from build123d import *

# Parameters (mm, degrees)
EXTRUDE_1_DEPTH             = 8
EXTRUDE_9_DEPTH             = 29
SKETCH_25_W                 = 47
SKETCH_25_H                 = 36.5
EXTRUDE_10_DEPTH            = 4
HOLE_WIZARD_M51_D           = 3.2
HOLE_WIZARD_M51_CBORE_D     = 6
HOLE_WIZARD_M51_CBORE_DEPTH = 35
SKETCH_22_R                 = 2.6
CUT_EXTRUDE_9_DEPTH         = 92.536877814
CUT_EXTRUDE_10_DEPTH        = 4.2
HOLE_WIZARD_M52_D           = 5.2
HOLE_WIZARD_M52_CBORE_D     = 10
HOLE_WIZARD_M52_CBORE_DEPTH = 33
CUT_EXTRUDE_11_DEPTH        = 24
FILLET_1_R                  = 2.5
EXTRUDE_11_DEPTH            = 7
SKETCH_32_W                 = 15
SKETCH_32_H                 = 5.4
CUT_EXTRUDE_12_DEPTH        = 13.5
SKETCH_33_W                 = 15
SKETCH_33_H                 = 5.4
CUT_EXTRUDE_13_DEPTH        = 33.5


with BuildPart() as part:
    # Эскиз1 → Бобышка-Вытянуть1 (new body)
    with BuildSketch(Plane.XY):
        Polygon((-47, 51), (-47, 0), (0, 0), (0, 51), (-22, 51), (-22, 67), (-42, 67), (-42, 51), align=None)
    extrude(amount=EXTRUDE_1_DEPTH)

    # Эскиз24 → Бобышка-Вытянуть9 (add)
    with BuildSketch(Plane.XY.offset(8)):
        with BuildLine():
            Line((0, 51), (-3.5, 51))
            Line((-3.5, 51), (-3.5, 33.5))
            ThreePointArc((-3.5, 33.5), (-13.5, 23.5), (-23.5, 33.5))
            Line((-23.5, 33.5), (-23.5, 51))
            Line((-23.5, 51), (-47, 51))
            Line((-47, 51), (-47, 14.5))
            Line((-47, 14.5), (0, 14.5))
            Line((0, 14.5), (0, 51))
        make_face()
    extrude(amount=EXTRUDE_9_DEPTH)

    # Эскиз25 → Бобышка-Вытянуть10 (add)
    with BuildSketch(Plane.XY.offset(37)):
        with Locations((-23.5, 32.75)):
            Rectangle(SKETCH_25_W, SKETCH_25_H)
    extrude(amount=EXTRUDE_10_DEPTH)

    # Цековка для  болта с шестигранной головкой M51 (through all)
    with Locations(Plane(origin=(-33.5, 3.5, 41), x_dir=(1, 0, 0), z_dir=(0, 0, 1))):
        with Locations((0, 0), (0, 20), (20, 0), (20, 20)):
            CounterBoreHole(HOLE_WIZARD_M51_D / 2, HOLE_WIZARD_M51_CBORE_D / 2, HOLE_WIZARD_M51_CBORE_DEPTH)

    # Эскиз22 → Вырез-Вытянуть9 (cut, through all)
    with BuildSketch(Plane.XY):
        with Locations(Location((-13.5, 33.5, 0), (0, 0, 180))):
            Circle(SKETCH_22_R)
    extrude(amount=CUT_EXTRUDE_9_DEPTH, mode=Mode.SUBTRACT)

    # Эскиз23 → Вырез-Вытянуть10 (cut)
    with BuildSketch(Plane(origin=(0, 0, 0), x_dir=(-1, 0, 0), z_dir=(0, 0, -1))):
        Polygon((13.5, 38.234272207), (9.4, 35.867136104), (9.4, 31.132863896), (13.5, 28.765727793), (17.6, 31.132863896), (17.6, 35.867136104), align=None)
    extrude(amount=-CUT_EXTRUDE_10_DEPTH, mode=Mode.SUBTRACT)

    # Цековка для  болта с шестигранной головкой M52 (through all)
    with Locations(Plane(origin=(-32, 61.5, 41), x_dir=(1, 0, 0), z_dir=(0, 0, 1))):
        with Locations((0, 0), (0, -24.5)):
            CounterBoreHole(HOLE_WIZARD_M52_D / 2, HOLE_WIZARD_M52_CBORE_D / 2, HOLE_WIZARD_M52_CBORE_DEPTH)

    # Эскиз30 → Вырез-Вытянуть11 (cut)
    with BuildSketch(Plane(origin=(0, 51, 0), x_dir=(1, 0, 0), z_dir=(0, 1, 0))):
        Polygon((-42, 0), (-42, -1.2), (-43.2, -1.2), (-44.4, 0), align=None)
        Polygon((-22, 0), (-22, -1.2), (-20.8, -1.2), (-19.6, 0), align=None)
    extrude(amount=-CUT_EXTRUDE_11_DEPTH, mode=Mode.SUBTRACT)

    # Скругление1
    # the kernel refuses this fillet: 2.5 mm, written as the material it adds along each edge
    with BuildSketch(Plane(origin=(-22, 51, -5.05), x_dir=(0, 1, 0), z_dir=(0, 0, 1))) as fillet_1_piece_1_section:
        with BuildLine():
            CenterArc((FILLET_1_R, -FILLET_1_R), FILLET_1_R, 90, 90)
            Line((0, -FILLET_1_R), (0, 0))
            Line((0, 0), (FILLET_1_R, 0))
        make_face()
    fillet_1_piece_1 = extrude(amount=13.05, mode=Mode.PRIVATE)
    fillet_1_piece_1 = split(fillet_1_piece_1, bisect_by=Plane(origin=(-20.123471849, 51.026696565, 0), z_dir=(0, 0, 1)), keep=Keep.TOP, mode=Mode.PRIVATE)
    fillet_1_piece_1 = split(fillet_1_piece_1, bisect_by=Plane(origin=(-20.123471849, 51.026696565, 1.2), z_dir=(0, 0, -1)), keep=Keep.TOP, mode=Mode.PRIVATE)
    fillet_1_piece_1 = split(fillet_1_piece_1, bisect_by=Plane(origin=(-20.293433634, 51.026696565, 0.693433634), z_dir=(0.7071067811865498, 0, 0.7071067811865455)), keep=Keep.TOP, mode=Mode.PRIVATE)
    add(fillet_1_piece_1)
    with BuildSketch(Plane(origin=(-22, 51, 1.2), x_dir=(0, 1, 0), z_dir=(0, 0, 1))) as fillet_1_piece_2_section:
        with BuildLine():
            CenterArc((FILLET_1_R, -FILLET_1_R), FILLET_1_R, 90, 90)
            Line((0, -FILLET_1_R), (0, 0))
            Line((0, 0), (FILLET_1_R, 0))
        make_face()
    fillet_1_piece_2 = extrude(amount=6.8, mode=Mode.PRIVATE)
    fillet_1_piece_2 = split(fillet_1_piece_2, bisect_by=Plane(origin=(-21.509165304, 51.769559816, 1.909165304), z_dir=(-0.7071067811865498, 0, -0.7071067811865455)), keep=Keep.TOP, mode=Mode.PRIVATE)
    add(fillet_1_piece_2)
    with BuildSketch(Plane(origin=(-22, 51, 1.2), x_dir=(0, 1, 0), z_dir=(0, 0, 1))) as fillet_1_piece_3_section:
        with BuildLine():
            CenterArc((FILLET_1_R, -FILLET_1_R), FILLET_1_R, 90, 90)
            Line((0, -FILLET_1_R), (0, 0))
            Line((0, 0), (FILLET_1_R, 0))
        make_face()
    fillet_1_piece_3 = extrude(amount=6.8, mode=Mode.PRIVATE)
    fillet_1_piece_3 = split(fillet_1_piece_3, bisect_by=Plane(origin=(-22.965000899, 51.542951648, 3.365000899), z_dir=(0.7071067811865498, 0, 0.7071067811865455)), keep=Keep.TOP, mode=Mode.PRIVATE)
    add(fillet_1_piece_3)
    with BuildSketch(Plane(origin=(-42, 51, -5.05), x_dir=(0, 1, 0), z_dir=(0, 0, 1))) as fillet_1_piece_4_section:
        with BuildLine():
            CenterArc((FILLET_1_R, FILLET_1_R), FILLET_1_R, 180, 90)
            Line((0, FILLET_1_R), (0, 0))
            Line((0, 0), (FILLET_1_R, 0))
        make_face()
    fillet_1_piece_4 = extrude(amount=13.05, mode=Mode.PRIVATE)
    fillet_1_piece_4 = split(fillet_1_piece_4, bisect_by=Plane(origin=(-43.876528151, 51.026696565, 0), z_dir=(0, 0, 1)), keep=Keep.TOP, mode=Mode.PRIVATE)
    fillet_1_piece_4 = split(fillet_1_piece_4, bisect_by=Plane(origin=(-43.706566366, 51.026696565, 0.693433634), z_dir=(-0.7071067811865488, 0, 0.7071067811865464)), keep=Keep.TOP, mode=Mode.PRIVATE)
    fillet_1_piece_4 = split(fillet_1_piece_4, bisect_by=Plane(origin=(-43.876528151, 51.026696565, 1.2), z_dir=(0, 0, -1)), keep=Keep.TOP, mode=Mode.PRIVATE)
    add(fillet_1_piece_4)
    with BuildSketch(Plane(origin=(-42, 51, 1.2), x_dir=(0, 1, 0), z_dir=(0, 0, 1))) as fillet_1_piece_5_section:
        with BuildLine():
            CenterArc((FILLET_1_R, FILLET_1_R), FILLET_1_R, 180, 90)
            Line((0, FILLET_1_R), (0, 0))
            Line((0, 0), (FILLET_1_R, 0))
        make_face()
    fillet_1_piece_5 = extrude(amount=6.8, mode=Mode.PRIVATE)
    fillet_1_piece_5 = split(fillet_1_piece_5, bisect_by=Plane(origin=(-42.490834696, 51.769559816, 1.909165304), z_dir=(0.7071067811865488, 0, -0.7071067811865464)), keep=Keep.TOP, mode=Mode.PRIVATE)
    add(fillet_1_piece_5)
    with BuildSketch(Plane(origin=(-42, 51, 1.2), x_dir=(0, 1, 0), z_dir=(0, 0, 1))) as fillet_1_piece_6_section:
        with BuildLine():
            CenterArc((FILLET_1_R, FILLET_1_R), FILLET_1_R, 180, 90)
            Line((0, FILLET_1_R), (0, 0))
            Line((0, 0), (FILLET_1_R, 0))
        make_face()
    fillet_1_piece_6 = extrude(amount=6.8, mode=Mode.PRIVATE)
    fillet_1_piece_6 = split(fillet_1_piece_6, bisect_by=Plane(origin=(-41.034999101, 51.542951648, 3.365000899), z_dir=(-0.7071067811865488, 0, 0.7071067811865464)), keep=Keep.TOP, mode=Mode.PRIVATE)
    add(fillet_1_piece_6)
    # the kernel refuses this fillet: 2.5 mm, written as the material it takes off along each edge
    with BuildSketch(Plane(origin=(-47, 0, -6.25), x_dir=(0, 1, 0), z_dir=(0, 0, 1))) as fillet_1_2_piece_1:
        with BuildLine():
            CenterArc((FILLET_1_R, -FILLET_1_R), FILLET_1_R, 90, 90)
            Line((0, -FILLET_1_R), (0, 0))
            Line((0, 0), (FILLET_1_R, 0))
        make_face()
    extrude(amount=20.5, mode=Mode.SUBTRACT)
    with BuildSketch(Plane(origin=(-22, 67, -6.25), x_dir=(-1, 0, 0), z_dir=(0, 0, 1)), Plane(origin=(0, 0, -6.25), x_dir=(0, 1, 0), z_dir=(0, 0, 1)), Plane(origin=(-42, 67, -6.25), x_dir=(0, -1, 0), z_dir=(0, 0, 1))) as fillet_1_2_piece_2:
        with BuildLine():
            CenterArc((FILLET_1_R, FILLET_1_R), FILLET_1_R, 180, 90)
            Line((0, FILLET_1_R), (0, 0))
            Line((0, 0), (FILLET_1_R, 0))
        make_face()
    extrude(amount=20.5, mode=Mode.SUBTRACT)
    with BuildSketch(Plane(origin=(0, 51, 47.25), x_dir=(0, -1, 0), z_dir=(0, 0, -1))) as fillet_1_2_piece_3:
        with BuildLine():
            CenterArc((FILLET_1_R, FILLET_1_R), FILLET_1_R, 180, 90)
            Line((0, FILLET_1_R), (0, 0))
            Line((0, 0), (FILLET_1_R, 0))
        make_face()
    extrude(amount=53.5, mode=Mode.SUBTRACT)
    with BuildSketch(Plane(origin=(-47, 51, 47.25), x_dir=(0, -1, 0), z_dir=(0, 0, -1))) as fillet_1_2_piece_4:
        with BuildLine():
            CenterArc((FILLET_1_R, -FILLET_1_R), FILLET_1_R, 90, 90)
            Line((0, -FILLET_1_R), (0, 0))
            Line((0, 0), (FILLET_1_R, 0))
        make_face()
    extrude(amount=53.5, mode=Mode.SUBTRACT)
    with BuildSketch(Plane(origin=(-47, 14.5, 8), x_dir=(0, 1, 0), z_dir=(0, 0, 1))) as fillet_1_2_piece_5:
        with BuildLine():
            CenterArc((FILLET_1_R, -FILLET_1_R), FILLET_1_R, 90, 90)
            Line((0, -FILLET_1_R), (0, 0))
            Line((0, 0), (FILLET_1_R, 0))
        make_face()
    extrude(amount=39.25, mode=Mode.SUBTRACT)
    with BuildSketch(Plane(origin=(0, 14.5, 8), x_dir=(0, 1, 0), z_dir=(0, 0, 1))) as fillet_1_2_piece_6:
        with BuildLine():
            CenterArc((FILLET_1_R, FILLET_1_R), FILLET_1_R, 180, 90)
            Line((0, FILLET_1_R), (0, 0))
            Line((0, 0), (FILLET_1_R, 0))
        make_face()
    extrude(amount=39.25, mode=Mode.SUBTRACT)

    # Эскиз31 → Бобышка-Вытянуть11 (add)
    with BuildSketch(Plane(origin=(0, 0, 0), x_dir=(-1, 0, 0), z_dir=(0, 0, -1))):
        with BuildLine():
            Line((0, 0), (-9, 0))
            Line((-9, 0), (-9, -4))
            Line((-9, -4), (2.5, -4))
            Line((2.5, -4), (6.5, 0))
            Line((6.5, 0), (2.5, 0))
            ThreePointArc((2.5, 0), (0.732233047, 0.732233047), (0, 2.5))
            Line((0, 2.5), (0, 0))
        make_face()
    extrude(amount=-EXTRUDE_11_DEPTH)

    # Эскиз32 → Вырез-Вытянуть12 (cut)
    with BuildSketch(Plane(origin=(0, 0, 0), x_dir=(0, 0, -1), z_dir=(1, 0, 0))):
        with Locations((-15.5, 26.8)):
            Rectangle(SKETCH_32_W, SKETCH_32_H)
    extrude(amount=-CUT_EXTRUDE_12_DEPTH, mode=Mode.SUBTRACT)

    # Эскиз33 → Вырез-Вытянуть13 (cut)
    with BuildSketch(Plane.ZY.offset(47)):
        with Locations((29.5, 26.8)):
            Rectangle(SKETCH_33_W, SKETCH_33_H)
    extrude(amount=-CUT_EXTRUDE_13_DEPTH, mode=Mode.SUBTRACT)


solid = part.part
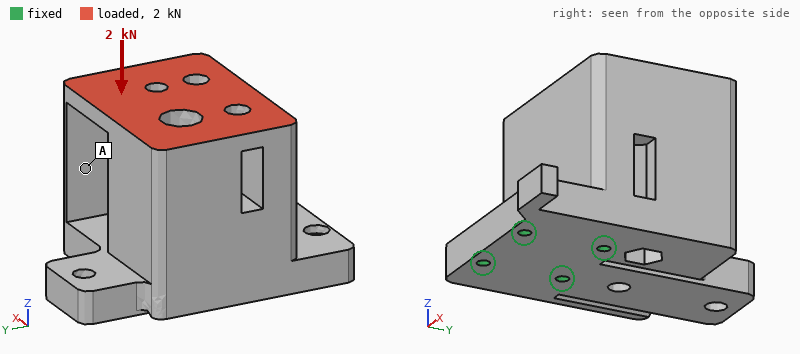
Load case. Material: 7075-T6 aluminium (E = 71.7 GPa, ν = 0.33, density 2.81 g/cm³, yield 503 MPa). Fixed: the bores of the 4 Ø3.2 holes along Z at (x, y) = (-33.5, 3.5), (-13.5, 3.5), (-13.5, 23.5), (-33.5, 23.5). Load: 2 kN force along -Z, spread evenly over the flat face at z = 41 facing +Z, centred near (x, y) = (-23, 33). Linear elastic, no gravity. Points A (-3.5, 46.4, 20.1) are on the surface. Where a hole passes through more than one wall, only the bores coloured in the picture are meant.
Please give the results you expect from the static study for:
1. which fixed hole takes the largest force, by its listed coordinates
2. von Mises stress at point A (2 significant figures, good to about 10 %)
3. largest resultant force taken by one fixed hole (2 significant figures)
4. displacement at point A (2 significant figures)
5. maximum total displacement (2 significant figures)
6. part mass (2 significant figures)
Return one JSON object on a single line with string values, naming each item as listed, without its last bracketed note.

{"which fixed hole takes the largest force, by its listed coordinates": "(-33.5, 23.5)", "von Mises stress at point A": "5.3 MPa", "largest resultant force taken by one fixed hole": "1.4 kN", "displacement at point A": "22 µm", "maximum total displacement": "36 µm", "part mass": "160 g"}
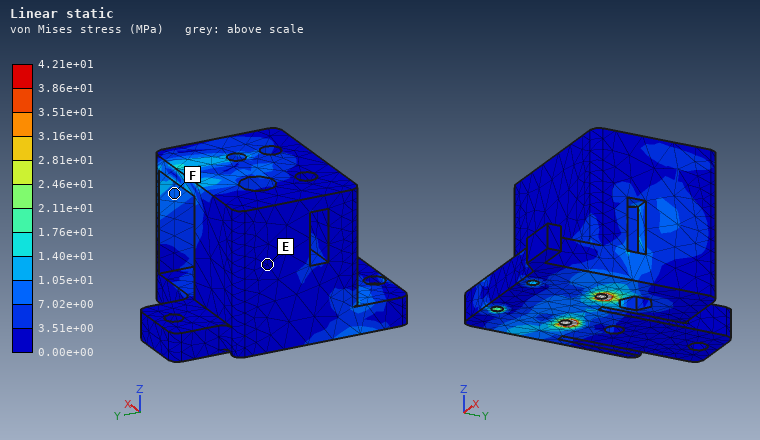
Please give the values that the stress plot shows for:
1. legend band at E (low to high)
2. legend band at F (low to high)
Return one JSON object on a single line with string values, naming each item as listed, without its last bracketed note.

{"legend band at E": "0.00e+00 to 3.51e+00 MPa", "legend band at F": "7.02e+00 to 1.05e+01 MPa"}
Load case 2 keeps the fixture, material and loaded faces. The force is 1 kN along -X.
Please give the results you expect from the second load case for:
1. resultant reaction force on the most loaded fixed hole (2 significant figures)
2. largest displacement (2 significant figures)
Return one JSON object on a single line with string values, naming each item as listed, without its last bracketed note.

{"resultant reaction force on the most loaded fixed hole": "1.4 kN", "largest displacement": "21 µm"}
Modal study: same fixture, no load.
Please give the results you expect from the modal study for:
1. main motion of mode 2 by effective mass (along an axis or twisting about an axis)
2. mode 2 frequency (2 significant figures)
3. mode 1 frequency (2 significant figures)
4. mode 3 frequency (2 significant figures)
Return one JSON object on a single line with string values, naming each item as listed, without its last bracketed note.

{"main motion of mode 2 by effective mass": "along X", "mode 2 frequency": "5300 Hz", "mode 1 frequency": "3300 Hz", "mode 3 frequency": "7900 Hz"}
